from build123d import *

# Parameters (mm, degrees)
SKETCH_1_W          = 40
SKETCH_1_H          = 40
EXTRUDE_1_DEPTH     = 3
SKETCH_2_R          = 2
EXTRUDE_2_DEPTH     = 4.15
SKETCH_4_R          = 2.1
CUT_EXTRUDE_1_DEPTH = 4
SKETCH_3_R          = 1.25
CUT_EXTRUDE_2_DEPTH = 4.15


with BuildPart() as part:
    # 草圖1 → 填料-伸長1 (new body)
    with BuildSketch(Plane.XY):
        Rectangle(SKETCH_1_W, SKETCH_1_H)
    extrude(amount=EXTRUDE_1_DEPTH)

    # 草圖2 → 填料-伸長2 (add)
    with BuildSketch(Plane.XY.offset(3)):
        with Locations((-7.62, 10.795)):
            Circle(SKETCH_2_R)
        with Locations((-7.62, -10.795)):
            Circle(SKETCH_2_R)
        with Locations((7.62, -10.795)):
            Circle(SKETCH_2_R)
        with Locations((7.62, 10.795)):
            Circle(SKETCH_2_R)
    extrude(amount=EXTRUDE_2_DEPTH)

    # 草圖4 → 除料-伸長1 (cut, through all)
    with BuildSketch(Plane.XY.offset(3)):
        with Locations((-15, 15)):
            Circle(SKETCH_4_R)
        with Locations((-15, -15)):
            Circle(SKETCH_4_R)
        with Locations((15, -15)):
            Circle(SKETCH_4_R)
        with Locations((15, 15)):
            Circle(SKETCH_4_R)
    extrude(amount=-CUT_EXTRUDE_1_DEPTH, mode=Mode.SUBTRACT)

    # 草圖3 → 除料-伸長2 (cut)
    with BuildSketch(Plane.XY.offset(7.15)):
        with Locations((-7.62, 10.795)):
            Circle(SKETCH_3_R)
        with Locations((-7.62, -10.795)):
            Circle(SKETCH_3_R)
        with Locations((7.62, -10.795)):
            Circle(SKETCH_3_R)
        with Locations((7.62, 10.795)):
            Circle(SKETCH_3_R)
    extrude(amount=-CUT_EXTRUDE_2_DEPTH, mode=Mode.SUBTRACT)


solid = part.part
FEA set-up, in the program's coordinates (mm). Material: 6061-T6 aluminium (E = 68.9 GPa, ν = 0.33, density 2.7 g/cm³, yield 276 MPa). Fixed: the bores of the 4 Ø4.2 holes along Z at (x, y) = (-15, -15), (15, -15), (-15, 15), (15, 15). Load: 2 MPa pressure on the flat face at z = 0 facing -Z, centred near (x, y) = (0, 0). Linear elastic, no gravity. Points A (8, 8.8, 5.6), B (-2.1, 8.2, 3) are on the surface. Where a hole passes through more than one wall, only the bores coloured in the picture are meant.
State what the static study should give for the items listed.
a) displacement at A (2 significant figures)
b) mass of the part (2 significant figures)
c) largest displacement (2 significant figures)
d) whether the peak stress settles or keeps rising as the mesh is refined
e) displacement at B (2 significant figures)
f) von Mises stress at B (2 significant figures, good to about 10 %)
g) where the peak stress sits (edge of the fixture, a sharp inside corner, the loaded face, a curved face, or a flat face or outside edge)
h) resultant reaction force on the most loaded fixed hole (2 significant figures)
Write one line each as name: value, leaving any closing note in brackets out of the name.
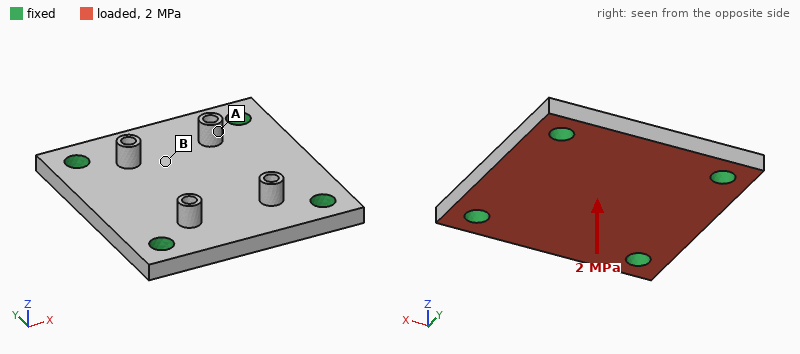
displacement at A: 32 µm
mass of the part: 13 g
largest displacement: 54 µm
whether the peak stress settles or keeps rising as the mesh is refined: keeps rising
displacement at B: 43 µm
von Mises stress at B: 45 MPa
where the peak stress sits: edge of the fixture
resultant reaction force on the most loaded fixed hole: 770 N
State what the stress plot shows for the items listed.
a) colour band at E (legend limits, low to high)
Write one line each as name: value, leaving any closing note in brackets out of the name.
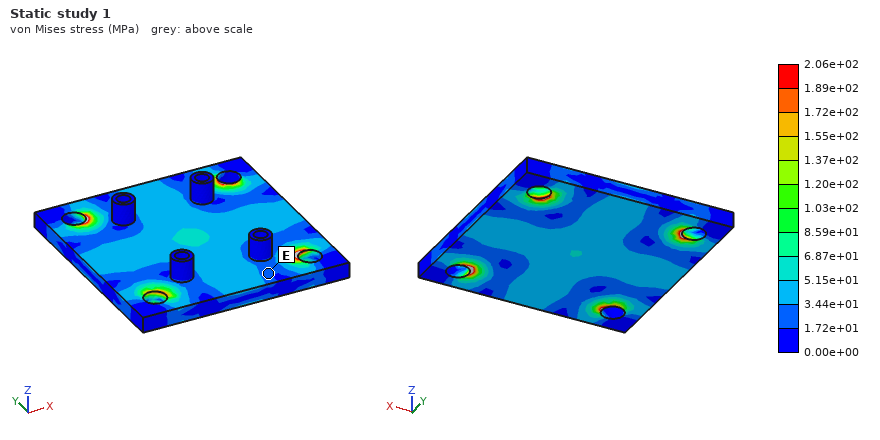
colour band at E: 1.72e+01 to 3.44e+01 MPa
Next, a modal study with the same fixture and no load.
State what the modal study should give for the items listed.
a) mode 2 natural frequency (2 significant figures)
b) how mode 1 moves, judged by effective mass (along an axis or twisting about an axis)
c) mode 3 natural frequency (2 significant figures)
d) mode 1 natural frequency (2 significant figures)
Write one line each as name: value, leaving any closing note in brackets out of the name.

mode 2 natural frequency: 20 kHz
how mode 1 moves, judged by effective mass: along Z
mode 3 natural frequency: 20 kHz
mode 1 natural frequency: 13 kHz
